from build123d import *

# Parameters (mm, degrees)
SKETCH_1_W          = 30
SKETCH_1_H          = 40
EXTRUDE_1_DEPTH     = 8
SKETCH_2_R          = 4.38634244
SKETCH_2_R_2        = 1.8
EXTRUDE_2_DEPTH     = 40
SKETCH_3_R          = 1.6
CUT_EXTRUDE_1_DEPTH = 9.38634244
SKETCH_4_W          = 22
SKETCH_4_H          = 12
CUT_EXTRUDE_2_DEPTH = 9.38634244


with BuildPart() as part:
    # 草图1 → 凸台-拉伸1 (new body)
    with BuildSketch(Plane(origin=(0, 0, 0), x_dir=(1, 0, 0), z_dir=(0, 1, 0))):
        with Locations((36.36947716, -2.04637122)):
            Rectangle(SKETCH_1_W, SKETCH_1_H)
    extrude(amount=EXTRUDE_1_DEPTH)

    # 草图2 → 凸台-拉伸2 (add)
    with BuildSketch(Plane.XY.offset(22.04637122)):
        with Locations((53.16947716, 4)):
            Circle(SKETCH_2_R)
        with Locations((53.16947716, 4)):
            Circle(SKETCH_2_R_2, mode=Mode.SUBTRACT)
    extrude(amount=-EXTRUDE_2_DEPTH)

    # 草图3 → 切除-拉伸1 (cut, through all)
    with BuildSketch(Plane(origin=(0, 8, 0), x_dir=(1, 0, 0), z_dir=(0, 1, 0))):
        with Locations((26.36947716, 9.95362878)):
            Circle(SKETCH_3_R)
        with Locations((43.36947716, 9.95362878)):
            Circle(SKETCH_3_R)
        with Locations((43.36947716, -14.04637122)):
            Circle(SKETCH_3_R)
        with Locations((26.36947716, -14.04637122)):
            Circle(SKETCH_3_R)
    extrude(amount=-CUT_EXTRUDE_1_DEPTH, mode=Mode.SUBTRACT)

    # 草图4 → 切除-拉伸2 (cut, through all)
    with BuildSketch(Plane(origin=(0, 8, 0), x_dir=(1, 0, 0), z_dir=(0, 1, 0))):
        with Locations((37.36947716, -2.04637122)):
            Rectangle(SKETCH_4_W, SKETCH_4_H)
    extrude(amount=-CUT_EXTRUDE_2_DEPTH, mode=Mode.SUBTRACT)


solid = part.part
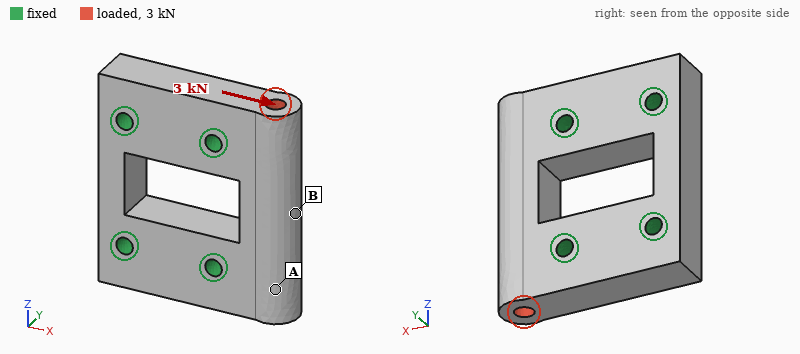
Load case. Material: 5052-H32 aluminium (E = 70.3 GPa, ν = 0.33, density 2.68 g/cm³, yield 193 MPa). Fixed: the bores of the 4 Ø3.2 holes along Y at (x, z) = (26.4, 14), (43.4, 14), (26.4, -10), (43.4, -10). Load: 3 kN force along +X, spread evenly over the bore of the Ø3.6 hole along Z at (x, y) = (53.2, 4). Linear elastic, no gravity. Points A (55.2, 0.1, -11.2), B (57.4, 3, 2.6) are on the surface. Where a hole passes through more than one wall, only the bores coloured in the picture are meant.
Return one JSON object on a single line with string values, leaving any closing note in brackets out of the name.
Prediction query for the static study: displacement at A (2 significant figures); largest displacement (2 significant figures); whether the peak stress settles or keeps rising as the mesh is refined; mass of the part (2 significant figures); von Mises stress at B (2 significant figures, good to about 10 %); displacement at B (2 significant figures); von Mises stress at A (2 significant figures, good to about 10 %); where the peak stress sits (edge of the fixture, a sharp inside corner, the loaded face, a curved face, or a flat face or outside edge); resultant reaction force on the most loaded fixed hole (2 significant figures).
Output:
{"displacement at A": "1.8 µm", "largest displacement": "5.1 µm", "whether the peak stress settles or keeps rising as the mesh is refined": "keeps rising", "mass of the part": "23 g", "von Mises stress at B": "14 MPa", "displacement at B": "4.8 µm", "von Mises stress at A": "4.5 MPa", "where the peak stress sits": "edge of the fixture", "resultant reaction force on the most loaded fixed hole": "1.3 kN"}
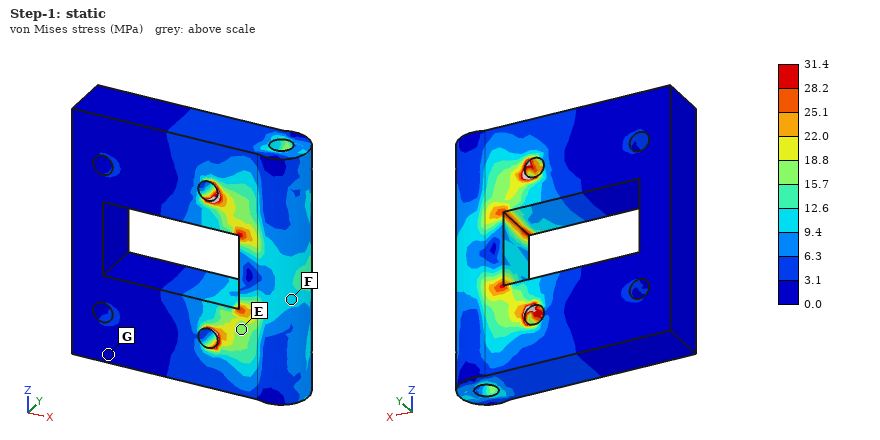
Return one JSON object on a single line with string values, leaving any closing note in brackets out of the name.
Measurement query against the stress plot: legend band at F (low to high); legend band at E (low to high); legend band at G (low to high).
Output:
{"legend band at F": "9.4 to 12.6 MPa", "legend band at E": "15.7 to 18.8 MPa", "legend band at G": "0.0 to 3.1 MPa"}
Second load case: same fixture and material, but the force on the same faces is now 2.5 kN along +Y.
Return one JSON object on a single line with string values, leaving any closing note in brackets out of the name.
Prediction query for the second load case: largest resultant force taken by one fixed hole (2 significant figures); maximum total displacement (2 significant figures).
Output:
{"largest resultant force taken by one fixed hole": "1.4 kN", "maximum total displacement": "28 µm"}
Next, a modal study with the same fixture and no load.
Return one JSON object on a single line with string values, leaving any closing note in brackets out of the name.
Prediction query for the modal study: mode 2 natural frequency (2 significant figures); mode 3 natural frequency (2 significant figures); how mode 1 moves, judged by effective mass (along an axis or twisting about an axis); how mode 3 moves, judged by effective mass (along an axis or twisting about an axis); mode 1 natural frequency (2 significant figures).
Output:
{"mode 2 natural frequency": "32 kHz", "mode 3 natural frequency": "36 kHz", "how mode 1 moves, judged by effective mass": "along Y", "how mode 3 moves, judged by effective mass": "along Z", "mode 1 natural frequency": "24 kHz"}
